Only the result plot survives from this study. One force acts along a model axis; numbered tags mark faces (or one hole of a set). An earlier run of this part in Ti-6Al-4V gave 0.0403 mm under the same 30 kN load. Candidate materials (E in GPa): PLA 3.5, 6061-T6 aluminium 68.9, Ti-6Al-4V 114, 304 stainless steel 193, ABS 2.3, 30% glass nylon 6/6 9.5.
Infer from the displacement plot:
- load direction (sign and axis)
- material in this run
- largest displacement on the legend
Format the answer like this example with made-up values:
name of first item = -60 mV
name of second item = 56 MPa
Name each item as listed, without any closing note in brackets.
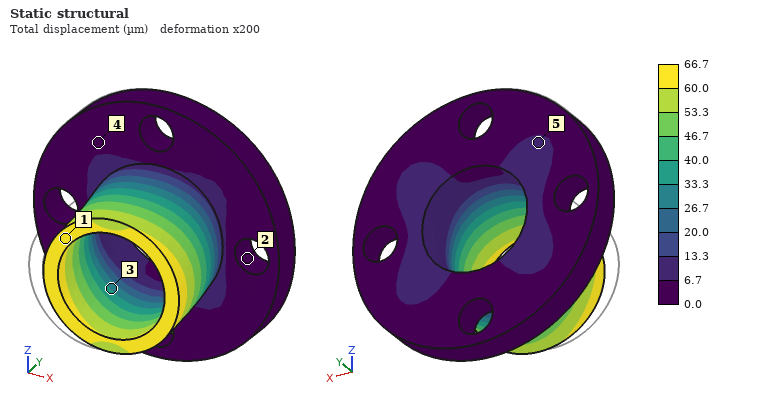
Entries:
load direction = +X
material in this run = 6061-T6 aluminium
largest displacement on the legend = 66.7 µm
